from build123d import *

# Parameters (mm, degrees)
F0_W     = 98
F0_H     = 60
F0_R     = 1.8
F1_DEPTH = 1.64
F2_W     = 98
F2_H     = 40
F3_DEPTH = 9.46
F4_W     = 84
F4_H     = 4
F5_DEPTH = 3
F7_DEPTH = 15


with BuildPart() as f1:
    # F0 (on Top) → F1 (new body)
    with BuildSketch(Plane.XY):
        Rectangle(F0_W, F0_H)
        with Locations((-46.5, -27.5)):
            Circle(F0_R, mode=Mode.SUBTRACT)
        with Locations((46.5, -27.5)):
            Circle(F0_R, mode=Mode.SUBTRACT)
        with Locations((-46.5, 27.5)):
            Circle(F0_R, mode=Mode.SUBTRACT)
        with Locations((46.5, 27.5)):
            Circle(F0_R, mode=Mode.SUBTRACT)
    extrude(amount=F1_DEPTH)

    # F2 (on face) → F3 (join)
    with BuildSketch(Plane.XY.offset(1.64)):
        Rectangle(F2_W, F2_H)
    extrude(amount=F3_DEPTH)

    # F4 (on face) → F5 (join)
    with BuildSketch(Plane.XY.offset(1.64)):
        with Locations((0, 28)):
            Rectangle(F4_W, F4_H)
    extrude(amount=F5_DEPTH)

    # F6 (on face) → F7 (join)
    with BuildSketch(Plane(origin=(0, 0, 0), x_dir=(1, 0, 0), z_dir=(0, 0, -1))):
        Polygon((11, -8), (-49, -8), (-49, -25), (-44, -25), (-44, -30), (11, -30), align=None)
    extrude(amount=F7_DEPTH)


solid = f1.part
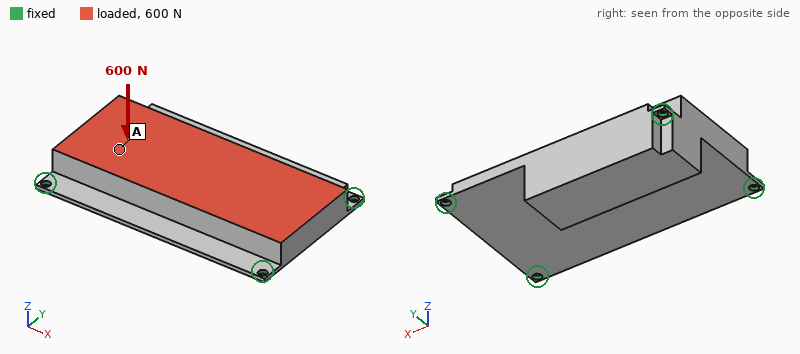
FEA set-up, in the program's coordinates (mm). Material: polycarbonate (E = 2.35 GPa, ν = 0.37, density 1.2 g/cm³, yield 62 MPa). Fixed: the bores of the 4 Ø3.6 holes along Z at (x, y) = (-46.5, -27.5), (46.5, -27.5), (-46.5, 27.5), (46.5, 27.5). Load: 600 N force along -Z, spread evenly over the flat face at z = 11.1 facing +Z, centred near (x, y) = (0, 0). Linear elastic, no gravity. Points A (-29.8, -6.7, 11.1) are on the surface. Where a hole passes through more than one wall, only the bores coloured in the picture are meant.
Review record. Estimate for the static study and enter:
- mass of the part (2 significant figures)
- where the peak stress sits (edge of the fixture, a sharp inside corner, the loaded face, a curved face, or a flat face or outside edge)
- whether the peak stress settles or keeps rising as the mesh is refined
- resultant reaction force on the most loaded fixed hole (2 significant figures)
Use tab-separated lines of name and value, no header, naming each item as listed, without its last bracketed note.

mass of the part	81 g
where the peak stress sits	edge of the fixture
whether the peak stress settles or keeps rising as the mesh is refined	keeps rising
resultant reaction force on the most loaded fixed hole	220 N
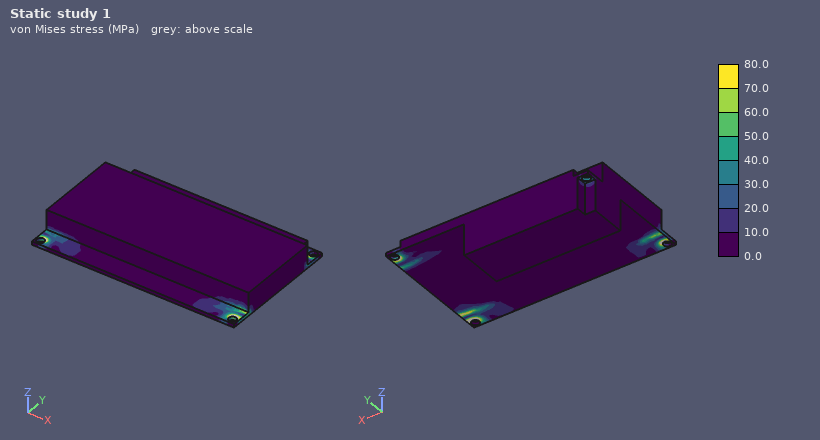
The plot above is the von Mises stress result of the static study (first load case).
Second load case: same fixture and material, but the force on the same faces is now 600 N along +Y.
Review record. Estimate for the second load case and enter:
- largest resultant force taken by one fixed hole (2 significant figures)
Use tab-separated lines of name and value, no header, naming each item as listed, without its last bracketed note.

largest resultant force taken by one fixed hole	180 N
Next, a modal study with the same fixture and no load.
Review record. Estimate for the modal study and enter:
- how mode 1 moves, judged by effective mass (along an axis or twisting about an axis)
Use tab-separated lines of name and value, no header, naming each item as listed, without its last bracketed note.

how mode 1 moves, judged by effective mass	along Z
